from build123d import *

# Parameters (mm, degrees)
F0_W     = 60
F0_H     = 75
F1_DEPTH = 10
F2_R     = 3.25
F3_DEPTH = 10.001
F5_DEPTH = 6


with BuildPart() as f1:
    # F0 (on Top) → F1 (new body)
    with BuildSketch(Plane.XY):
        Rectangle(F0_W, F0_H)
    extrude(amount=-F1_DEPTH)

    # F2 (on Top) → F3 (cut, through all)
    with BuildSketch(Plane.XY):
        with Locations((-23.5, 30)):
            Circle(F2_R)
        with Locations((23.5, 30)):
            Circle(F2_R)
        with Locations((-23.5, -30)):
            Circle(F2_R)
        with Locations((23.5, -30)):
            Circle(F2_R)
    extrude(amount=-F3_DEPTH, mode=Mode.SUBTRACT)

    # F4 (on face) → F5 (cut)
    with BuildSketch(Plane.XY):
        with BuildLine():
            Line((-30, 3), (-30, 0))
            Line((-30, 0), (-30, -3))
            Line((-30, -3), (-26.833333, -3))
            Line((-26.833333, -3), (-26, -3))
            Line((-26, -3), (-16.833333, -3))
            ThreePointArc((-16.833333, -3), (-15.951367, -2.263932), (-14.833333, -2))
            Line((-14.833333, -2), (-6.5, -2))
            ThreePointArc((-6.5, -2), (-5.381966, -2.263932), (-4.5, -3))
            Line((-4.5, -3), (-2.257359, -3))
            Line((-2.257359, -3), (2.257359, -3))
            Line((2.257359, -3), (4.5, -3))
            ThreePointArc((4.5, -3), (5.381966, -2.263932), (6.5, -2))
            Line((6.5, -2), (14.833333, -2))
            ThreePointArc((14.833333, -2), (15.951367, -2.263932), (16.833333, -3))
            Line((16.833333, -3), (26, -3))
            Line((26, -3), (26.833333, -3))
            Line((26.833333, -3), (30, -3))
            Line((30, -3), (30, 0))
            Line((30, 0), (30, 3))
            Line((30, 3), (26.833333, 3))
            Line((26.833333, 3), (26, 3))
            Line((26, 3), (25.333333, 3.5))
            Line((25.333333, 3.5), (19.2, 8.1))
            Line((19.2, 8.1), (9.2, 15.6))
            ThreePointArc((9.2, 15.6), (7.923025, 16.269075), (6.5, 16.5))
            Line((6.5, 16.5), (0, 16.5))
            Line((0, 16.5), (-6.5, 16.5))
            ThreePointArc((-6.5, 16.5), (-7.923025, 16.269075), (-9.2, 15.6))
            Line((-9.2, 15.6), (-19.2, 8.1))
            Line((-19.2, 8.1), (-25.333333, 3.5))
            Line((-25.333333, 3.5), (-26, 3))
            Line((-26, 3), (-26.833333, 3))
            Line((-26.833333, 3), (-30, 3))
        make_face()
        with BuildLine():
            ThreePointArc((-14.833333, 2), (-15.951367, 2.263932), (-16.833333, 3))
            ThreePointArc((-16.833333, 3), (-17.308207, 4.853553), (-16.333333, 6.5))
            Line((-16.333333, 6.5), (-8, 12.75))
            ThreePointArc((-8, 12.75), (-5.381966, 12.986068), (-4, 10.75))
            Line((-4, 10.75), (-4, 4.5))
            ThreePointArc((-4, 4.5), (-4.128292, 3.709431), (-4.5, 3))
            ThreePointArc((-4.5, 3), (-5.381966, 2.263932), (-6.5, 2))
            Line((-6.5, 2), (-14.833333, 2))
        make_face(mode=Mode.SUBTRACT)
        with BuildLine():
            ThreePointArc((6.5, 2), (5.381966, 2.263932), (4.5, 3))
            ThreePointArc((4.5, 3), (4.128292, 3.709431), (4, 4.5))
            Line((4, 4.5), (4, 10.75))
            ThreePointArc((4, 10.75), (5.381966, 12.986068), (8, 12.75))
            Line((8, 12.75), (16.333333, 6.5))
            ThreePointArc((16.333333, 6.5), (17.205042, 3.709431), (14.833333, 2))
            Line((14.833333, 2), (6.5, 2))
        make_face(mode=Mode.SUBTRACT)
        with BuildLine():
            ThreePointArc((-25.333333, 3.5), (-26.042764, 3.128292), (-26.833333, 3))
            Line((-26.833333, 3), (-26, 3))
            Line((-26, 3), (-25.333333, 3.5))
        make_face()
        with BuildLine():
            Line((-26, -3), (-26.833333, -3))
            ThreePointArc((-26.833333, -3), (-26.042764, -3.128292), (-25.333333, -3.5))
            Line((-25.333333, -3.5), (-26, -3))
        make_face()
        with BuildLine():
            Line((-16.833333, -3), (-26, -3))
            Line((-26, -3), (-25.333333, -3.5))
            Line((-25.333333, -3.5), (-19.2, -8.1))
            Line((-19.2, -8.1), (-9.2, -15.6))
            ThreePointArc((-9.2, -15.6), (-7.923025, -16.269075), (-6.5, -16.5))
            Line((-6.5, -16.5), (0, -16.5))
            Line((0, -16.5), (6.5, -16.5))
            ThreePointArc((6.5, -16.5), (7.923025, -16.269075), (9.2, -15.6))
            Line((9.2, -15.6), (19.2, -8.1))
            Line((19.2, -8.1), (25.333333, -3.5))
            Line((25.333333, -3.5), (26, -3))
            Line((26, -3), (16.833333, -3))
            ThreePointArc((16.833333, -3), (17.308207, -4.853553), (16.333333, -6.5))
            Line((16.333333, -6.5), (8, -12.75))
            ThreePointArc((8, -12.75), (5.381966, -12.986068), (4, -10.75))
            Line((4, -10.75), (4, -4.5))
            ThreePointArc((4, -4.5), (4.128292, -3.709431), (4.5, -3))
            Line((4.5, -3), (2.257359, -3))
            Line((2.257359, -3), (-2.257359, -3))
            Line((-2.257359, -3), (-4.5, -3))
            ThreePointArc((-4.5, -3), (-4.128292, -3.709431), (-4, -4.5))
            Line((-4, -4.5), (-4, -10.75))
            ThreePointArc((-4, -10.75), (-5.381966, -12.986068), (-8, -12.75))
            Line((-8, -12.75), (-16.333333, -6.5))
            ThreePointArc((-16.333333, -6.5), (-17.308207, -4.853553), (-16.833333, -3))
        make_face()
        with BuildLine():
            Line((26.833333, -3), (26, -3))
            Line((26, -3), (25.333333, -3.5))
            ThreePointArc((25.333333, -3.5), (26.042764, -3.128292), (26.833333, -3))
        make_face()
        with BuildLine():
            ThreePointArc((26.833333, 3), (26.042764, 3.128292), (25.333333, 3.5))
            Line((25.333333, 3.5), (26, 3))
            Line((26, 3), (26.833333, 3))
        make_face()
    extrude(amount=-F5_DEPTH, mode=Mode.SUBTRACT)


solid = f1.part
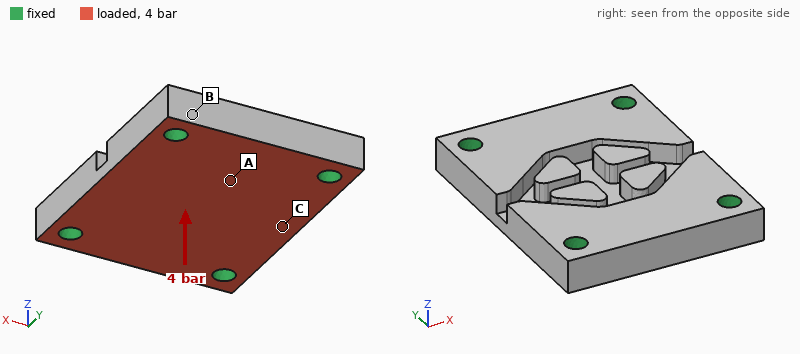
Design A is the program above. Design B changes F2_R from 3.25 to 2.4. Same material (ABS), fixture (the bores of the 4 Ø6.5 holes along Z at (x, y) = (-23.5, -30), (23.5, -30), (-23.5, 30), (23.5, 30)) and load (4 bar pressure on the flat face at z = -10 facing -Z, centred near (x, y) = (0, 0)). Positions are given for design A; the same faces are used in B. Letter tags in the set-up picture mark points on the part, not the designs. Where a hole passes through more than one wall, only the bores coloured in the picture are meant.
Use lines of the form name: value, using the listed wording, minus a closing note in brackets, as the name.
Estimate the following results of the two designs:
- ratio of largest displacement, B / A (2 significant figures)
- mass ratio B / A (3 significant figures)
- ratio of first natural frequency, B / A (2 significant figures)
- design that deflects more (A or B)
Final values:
ratio of largest displacement, B / A: 1.1
mass ratio B / A: 1.02
ratio of first natural frequency, B / A: 0.92
design that deflects more: B
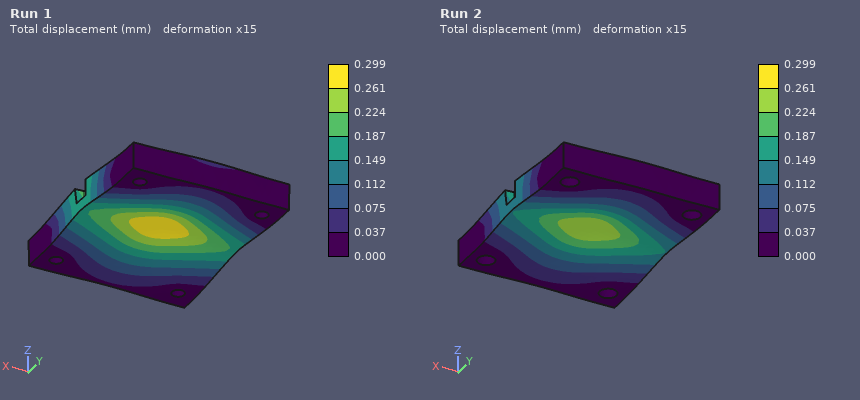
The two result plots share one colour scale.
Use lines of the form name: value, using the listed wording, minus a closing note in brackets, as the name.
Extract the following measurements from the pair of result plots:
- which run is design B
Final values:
which run is design B: Run 1
